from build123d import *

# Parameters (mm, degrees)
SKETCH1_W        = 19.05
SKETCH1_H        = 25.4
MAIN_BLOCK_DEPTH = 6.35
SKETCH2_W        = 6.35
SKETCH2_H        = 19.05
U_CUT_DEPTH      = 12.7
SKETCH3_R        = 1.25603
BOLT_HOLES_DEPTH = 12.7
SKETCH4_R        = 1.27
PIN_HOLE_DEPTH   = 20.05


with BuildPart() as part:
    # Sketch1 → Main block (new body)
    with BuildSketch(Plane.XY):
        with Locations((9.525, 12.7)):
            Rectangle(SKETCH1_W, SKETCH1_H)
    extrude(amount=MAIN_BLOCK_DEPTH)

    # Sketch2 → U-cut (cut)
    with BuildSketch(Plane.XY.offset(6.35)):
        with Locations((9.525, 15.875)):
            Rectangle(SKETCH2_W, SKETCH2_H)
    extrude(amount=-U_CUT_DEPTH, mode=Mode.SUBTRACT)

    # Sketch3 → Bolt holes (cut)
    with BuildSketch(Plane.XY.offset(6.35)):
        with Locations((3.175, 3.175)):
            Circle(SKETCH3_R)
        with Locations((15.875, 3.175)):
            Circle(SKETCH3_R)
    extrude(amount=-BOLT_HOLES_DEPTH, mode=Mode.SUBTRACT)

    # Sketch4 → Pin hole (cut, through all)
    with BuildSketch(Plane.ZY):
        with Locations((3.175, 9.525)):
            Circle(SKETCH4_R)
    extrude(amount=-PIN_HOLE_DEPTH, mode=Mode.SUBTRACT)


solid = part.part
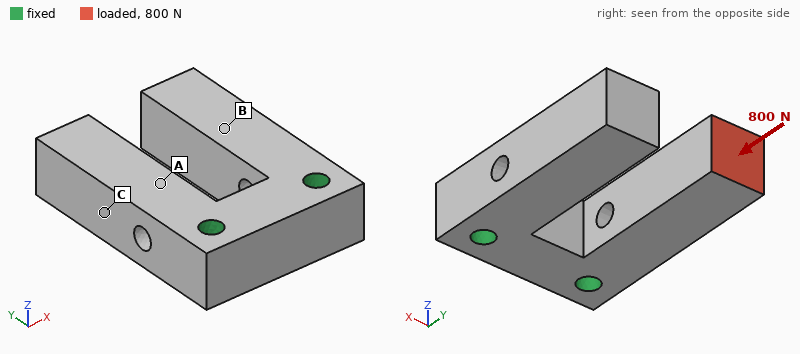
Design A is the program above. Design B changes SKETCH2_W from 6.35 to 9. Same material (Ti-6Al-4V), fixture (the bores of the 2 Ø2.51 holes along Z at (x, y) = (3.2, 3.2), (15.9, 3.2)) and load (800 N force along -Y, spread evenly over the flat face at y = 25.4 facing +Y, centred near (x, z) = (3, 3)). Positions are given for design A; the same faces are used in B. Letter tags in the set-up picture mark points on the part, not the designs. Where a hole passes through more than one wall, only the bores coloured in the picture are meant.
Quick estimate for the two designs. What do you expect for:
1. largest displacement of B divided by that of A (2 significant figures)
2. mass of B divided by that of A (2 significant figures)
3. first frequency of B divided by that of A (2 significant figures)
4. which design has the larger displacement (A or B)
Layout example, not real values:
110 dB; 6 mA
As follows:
1.5; 0.86; 0.86; B
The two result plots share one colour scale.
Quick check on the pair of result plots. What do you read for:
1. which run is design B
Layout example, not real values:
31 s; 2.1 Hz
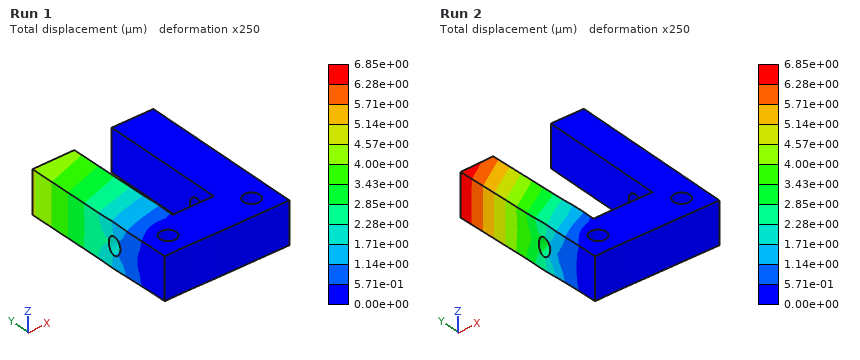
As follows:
Run 2
